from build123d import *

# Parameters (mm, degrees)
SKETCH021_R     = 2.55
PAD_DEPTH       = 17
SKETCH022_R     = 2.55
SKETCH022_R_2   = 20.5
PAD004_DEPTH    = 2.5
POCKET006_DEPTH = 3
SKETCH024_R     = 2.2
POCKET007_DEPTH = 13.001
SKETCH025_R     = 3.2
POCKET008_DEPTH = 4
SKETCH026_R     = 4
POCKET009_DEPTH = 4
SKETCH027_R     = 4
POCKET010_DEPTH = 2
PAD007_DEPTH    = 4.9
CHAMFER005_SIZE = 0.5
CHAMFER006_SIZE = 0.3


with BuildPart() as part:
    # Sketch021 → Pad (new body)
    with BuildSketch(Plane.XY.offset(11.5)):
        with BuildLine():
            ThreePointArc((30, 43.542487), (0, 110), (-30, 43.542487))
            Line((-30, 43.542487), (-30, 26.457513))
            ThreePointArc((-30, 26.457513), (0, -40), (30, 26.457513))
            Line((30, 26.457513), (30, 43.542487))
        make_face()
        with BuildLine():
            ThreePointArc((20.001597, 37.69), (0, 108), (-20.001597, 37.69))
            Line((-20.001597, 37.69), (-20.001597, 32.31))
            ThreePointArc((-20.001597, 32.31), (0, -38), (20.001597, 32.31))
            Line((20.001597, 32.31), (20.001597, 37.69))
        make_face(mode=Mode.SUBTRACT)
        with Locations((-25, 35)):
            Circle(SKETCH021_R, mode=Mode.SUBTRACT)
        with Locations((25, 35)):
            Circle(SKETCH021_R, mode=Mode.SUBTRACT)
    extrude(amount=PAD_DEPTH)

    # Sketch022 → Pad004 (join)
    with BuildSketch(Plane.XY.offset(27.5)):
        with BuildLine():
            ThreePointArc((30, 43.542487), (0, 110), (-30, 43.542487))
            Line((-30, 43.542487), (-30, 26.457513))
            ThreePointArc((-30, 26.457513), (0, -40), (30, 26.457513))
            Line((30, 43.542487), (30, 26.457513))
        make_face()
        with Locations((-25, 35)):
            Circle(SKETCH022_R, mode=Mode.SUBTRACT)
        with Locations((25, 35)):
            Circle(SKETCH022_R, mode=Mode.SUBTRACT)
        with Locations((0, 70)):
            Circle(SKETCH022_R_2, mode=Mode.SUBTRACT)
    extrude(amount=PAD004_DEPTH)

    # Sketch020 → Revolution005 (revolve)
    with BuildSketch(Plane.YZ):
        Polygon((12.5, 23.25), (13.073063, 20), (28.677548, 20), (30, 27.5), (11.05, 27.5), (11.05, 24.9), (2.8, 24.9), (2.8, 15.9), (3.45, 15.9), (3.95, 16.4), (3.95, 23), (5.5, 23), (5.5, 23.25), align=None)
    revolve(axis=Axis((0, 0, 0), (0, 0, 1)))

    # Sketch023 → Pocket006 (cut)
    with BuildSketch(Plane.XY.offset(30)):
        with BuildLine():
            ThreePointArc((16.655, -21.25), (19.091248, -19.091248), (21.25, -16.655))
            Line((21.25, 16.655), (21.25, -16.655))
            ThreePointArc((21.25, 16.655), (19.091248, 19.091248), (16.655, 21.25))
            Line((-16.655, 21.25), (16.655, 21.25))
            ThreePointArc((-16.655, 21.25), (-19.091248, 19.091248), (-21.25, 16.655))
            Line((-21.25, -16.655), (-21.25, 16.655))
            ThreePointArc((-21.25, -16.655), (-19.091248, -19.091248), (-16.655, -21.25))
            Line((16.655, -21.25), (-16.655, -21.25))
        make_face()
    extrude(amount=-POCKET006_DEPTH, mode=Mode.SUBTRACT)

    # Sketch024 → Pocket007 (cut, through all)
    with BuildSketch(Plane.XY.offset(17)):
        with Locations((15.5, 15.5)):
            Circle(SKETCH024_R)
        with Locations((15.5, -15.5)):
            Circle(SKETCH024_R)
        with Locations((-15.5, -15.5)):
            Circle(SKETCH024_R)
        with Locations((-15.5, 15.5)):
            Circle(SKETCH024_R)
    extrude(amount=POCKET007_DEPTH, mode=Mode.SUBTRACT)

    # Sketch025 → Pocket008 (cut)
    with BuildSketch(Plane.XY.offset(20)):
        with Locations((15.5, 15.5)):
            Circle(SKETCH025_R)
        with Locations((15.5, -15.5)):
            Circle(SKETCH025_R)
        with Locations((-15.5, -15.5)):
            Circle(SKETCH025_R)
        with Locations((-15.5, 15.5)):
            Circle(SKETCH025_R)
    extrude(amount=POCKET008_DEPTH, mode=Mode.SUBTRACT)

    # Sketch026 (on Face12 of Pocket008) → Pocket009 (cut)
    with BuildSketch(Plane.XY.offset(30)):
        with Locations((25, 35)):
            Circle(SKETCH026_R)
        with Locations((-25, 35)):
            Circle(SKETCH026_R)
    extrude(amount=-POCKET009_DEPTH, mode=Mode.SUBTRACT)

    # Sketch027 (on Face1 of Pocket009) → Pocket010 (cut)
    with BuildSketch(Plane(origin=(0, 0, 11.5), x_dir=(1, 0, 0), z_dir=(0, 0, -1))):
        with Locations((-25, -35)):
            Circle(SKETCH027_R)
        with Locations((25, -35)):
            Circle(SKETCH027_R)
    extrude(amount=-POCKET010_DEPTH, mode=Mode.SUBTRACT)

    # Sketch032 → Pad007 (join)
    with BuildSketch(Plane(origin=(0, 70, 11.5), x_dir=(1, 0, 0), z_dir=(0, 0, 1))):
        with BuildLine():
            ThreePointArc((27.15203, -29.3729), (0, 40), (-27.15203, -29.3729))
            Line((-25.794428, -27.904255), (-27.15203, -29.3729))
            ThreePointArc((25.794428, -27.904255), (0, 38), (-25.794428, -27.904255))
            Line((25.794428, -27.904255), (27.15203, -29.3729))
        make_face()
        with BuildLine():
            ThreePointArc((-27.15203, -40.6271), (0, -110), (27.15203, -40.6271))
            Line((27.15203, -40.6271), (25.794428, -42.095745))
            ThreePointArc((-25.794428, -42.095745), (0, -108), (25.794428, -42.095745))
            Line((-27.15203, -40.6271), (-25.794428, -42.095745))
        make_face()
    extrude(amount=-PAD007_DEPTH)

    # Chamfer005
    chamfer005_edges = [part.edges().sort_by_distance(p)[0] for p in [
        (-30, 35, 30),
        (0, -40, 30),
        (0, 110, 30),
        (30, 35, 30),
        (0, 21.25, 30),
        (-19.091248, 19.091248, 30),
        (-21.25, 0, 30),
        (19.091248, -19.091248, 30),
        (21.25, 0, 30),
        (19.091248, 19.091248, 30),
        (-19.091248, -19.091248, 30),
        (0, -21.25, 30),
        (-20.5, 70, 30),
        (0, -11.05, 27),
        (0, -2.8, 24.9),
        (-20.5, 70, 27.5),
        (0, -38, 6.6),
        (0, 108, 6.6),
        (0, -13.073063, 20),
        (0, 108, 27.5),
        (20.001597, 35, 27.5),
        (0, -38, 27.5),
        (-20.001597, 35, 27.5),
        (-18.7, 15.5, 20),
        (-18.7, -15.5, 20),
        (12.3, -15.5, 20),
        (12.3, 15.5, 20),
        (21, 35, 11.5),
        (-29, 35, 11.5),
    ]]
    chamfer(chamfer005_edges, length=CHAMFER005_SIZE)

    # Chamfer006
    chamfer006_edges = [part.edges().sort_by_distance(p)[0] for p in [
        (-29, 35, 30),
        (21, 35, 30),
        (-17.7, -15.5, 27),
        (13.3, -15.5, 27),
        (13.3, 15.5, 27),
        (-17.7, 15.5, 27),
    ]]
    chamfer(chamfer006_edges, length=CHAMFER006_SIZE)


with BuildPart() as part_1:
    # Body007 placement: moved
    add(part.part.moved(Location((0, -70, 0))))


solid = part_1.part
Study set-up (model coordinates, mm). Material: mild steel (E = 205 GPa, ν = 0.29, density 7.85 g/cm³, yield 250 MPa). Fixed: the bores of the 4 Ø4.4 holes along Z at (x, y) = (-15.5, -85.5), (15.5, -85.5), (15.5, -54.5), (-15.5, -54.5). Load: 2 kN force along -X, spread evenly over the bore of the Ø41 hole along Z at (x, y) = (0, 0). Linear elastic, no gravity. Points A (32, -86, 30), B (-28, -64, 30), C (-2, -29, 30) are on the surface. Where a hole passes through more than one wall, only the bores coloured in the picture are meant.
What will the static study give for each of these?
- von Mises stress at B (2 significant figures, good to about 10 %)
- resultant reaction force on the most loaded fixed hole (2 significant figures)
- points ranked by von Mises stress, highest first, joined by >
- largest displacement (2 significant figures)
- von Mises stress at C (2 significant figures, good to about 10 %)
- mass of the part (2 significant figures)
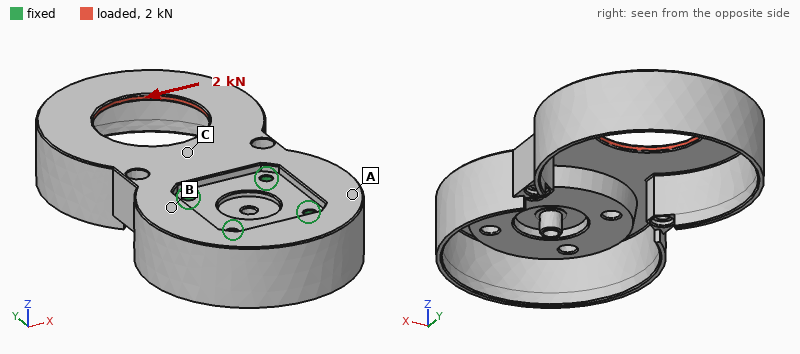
15 MPa
2.3 kN
C > B > A
88 µm
53 MPa
400 g
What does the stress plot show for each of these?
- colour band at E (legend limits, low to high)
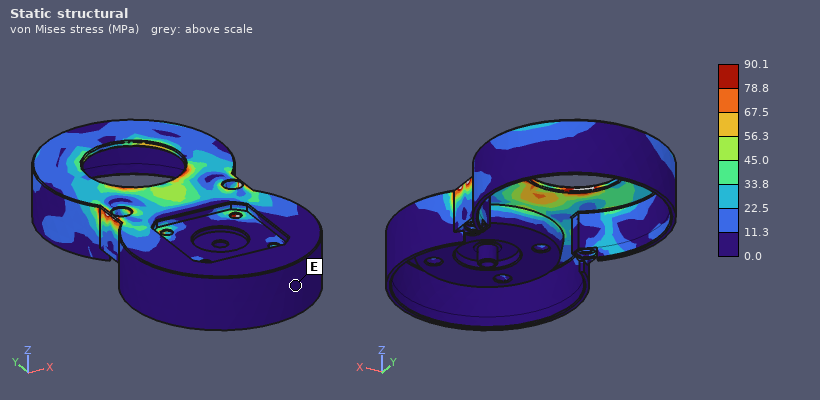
0.0 to 11.3 MPa
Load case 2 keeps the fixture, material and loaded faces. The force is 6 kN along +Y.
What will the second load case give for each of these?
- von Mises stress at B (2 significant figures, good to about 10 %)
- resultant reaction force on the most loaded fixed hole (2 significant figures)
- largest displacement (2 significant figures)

24 MPa
2.5 kN
0.11 mm
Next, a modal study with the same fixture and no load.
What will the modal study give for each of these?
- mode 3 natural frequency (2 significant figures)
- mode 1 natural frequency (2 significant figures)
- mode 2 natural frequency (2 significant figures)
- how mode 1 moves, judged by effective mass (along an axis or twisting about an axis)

1900 Hz
460 Hz
790 Hz
along Z
